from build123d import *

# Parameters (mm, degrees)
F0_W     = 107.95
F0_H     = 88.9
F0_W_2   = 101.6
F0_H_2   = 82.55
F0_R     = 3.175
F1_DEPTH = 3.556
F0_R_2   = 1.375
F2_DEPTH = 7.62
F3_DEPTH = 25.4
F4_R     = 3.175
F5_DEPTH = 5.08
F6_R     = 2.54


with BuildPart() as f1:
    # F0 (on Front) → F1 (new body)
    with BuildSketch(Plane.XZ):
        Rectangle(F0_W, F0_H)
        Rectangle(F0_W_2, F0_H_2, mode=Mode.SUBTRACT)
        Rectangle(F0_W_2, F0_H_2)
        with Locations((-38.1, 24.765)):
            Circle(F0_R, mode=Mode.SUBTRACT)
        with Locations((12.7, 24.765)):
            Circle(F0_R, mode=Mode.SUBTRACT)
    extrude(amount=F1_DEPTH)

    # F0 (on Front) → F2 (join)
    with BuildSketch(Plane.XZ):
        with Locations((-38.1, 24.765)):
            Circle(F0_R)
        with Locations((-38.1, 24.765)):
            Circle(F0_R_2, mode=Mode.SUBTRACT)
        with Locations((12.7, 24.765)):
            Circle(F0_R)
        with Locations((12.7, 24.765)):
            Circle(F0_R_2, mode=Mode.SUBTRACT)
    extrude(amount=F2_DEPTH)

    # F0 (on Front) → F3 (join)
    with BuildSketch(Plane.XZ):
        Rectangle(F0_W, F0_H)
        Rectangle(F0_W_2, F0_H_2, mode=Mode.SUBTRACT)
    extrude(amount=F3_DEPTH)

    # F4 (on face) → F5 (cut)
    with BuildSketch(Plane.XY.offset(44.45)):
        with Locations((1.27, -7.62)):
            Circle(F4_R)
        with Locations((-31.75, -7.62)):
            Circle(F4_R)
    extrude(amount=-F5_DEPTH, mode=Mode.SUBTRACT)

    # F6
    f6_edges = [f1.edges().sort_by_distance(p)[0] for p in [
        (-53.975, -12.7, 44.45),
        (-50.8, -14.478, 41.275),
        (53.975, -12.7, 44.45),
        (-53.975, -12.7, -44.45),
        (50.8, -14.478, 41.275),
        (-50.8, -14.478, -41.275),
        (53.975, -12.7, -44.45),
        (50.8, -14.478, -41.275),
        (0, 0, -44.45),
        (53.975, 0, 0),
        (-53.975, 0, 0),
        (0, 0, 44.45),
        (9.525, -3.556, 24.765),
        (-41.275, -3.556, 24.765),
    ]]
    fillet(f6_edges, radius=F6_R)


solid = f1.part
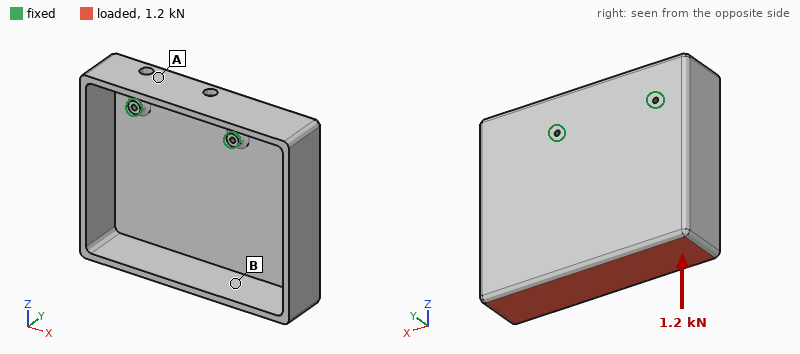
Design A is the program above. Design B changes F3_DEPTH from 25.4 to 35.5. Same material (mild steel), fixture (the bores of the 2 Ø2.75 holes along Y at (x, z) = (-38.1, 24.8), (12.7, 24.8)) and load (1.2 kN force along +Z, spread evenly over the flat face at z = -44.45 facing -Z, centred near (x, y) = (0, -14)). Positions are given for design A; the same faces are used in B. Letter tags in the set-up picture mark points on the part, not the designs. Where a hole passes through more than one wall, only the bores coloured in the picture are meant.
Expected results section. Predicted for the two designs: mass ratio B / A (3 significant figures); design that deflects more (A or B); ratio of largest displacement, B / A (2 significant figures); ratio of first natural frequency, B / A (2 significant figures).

1.20
B
1.4
0.89
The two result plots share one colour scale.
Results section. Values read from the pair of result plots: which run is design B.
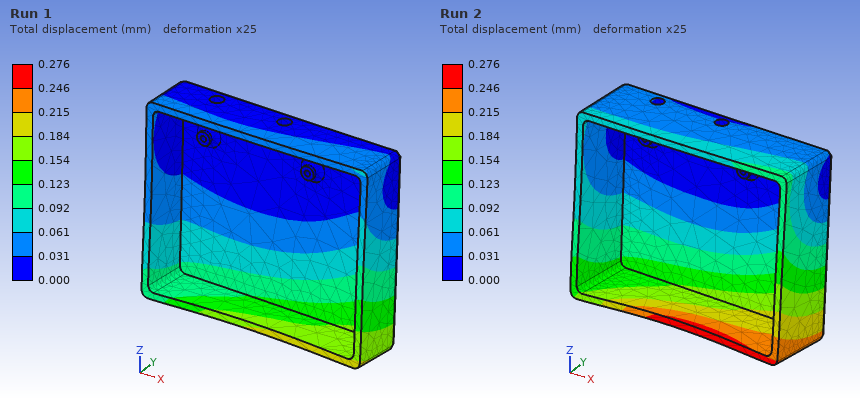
Run 2
